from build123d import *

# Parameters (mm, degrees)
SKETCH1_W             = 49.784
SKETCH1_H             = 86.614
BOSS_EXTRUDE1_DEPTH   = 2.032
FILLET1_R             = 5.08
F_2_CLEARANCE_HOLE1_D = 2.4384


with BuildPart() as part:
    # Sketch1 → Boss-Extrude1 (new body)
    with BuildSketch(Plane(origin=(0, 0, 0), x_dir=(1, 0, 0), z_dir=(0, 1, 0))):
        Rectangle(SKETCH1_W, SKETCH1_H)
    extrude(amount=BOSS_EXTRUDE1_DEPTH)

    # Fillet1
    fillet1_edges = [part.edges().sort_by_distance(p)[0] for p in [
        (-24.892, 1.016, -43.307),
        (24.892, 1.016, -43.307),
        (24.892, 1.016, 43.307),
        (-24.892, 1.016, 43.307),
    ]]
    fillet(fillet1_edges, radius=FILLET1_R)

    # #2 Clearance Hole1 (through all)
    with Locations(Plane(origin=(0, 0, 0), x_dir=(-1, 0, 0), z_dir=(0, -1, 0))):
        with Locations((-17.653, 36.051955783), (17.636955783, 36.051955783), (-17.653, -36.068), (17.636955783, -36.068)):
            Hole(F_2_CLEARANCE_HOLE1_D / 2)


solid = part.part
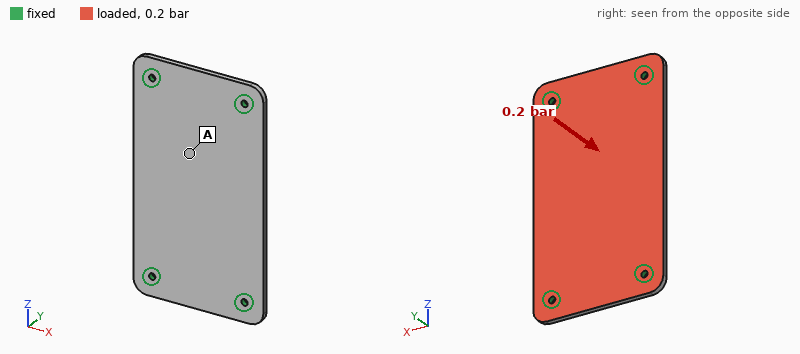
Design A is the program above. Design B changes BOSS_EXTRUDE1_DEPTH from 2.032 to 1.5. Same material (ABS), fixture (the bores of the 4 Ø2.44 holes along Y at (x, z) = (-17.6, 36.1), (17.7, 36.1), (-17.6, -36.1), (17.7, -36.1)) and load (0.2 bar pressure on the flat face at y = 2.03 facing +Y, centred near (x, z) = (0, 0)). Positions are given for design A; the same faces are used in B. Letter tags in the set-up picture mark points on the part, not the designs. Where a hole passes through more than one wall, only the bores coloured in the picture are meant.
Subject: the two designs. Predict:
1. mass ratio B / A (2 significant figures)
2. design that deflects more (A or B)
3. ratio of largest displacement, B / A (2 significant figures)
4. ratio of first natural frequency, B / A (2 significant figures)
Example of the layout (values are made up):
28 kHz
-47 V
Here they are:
0.74
B
2.4
0.75
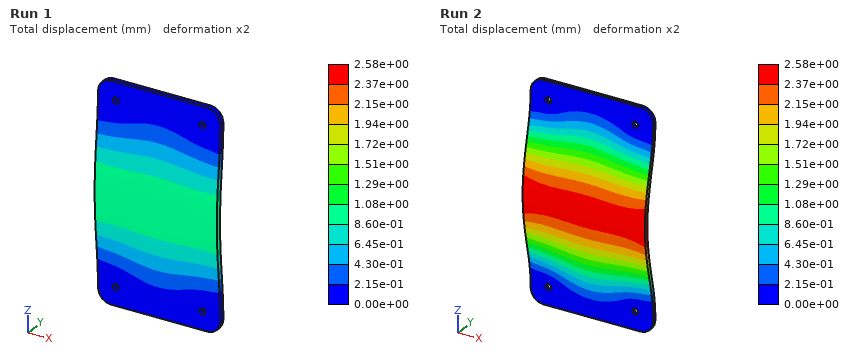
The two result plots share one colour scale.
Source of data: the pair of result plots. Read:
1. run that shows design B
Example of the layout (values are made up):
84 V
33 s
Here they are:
Run 2
